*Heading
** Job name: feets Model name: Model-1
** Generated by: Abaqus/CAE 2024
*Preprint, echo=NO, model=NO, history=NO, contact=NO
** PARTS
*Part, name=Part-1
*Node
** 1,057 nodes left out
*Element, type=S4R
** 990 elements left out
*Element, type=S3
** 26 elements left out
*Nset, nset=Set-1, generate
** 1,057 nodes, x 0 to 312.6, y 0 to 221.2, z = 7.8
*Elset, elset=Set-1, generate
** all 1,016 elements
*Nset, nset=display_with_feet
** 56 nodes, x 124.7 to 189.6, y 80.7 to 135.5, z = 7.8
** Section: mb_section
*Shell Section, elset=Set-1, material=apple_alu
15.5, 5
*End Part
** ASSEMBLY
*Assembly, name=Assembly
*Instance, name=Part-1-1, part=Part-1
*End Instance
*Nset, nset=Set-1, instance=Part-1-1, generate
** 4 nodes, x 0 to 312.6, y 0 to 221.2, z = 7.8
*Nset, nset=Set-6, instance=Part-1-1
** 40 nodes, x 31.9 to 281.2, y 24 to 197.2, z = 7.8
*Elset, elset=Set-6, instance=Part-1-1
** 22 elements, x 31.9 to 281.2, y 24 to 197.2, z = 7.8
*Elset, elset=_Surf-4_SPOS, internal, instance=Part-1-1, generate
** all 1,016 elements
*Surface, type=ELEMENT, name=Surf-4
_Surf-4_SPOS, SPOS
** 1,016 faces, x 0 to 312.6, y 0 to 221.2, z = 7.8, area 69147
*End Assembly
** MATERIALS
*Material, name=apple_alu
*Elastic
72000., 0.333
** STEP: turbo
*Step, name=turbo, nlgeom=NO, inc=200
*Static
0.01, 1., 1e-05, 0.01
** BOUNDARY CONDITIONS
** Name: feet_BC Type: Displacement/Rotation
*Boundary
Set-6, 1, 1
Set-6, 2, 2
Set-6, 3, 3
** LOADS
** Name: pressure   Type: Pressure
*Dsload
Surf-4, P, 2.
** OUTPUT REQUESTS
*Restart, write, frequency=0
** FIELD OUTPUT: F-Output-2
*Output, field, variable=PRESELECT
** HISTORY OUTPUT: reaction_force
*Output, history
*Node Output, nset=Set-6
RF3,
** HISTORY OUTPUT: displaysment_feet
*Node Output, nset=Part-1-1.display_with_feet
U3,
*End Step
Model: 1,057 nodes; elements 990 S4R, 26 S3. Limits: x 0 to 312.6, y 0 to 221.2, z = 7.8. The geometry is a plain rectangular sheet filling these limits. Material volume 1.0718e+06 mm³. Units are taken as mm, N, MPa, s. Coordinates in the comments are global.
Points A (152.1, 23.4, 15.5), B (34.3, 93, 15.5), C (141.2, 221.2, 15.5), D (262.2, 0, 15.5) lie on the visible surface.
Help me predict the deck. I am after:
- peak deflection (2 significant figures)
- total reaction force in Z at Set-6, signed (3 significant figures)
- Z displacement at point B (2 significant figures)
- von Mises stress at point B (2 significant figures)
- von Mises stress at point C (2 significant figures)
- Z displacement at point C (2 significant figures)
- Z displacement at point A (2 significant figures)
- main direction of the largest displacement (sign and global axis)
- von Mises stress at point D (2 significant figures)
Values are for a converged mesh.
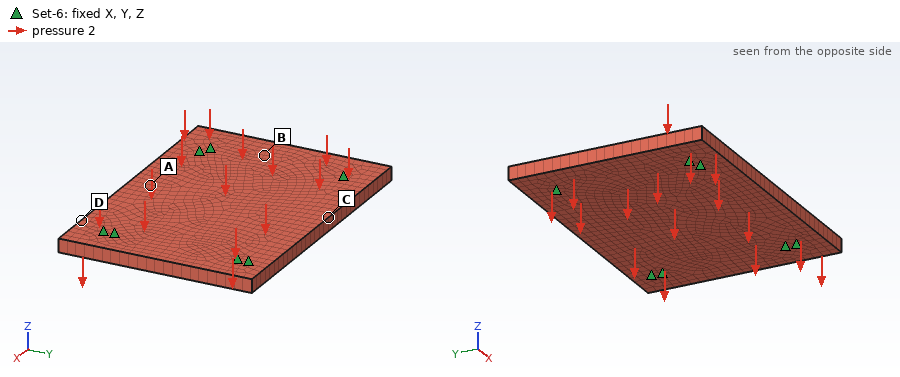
0.95 mm
1.38e+05 N
-0.17 mm
69 MPa
130 MPa
-0.80 mm
-0.84 mm
-Z
110 MPa
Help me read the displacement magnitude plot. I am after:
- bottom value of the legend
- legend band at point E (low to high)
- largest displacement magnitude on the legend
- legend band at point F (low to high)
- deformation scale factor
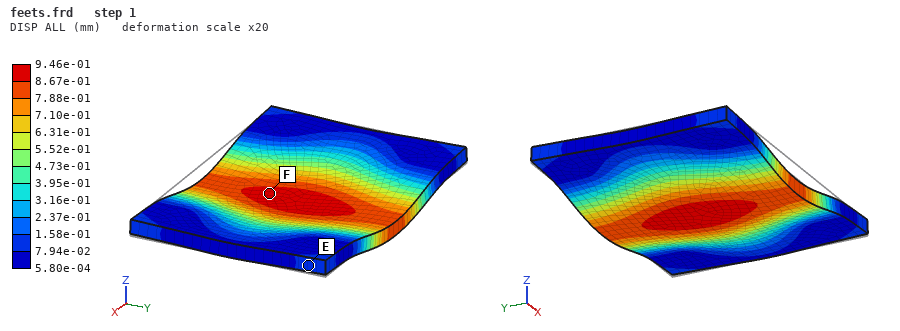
5.80e-04 mm
7.94e-02 to 1.58e-01 mm
9.46e-01 mm
8.67e-01 to 9.46e-01 mm
20
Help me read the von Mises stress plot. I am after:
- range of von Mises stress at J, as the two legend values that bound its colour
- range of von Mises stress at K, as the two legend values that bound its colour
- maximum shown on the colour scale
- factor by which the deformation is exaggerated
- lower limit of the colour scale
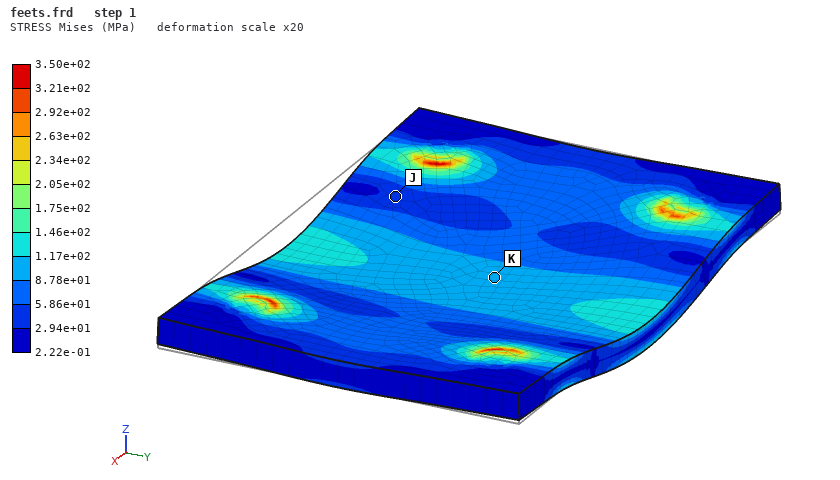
2.94e+01 to 5.86e+01 MPa
8.78e+01 to 1.17e+02 MPa
3.50e+02 MPa
20
2.22e-01 MPa
